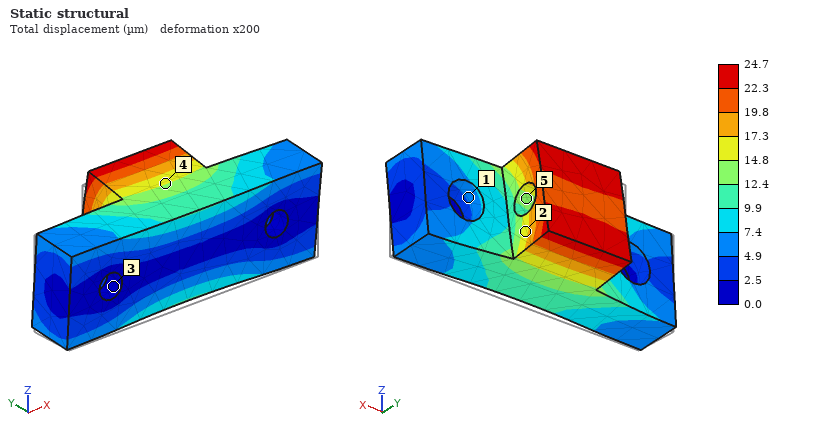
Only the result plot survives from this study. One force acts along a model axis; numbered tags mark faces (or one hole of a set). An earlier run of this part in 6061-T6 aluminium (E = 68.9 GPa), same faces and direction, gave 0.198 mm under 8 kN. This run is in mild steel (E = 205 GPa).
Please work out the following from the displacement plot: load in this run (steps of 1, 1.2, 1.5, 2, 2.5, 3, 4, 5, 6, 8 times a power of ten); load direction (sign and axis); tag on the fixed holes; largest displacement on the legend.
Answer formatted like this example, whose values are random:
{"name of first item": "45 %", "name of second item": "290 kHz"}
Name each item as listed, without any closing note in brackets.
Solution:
{"load in this run": "3 kN", "load direction": "+Z", "tag on the fixed holes": "3", "largest displacement on the legend": "24.7 µm"}
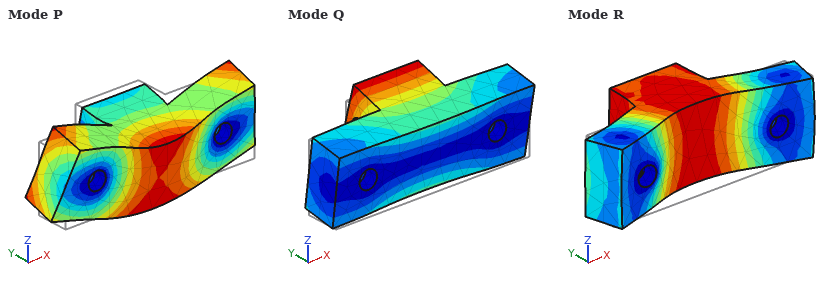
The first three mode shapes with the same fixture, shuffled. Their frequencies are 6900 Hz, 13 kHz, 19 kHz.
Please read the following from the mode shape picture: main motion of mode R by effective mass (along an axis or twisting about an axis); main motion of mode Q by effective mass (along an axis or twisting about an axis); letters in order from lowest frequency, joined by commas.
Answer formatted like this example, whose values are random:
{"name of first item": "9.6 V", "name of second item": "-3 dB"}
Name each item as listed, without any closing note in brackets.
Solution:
{"main motion of mode R by effective mass": "along Y", "main motion of mode Q by effective mass": "along Z", "letters in order from lowest frequency, joined by commas": "Q, R, P"}
